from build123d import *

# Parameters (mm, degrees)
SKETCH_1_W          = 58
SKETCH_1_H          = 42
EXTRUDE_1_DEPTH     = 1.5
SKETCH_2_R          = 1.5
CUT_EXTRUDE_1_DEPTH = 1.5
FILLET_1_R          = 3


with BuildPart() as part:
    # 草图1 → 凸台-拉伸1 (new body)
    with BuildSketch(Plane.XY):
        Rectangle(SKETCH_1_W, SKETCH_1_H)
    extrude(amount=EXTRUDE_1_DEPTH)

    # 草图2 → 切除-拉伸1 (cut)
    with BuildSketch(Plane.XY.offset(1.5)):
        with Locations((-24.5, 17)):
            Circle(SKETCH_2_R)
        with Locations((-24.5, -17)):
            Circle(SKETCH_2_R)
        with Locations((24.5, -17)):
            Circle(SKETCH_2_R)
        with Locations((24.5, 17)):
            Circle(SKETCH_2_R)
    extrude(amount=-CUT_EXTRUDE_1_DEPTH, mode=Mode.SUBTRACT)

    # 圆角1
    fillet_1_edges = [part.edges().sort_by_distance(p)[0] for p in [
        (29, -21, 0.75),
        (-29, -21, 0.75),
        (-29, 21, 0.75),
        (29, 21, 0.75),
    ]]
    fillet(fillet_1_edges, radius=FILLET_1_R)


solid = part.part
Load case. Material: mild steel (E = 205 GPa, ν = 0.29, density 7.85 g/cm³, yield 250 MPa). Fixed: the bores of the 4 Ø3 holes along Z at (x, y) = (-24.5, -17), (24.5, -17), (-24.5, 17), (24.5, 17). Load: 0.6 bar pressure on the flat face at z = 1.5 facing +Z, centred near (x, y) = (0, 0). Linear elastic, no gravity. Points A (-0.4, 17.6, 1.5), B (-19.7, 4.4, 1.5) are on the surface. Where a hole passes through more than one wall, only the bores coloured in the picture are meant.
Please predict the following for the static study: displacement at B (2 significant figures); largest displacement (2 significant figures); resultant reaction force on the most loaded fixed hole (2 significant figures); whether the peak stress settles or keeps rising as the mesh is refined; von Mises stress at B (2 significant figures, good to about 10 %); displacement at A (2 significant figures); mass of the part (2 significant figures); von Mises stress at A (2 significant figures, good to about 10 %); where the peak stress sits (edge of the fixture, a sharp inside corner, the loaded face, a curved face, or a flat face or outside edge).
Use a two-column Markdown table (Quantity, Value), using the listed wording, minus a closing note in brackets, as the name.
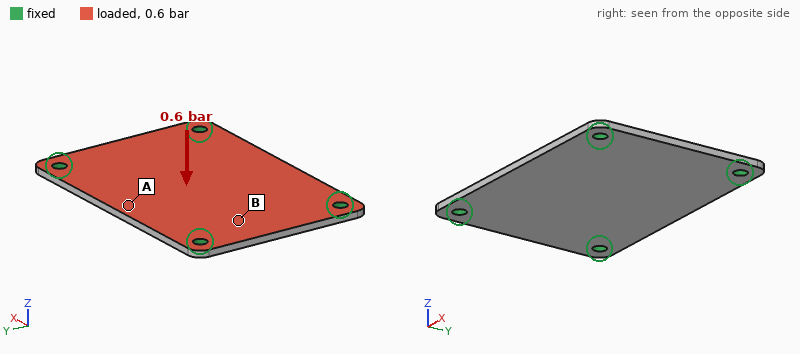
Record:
| Quantity | Value |
|---|---|
| displacement at B | 8.1 µm |
| largest displacement | 22 µm |
| resultant reaction force on the most loaded fixed hole | 36 N |
| whether the peak stress settles or keeps rising as the mesh is refined | keeps rising |
| von Mises stress at B | 10 MPa |
| displacement at A | 18 µm |
| mass of the part | 28 g |
| von Mises stress at A | 18 MPa |
| where the peak stress sits | edge of the fixture |
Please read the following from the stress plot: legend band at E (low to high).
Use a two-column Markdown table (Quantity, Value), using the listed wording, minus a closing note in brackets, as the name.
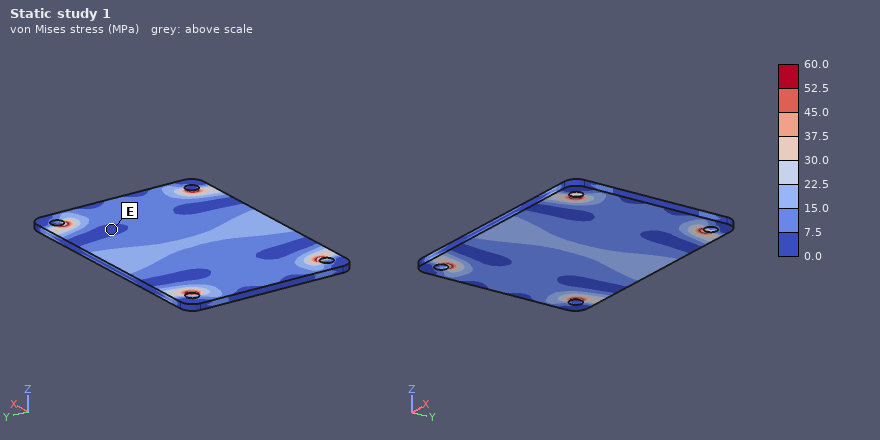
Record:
| Quantity | Value |
|---|---|
| legend band at E | 0.0 to 7.5 MPa |
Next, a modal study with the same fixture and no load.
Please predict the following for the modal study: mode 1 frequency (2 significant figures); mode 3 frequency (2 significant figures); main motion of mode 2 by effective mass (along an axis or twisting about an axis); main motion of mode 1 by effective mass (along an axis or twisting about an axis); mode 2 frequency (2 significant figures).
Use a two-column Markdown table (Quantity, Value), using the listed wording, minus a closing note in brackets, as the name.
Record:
| Quantity | Value |
|---|---|
| mode 1 frequency | 2900 Hz |
| mode 3 frequency | 6500 Hz |
| main motion of mode 2 by effective mass | twisting about X |
| main motion of mode 1 by effective mass | along Z |
| mode 2 frequency | 4300 Hz |
